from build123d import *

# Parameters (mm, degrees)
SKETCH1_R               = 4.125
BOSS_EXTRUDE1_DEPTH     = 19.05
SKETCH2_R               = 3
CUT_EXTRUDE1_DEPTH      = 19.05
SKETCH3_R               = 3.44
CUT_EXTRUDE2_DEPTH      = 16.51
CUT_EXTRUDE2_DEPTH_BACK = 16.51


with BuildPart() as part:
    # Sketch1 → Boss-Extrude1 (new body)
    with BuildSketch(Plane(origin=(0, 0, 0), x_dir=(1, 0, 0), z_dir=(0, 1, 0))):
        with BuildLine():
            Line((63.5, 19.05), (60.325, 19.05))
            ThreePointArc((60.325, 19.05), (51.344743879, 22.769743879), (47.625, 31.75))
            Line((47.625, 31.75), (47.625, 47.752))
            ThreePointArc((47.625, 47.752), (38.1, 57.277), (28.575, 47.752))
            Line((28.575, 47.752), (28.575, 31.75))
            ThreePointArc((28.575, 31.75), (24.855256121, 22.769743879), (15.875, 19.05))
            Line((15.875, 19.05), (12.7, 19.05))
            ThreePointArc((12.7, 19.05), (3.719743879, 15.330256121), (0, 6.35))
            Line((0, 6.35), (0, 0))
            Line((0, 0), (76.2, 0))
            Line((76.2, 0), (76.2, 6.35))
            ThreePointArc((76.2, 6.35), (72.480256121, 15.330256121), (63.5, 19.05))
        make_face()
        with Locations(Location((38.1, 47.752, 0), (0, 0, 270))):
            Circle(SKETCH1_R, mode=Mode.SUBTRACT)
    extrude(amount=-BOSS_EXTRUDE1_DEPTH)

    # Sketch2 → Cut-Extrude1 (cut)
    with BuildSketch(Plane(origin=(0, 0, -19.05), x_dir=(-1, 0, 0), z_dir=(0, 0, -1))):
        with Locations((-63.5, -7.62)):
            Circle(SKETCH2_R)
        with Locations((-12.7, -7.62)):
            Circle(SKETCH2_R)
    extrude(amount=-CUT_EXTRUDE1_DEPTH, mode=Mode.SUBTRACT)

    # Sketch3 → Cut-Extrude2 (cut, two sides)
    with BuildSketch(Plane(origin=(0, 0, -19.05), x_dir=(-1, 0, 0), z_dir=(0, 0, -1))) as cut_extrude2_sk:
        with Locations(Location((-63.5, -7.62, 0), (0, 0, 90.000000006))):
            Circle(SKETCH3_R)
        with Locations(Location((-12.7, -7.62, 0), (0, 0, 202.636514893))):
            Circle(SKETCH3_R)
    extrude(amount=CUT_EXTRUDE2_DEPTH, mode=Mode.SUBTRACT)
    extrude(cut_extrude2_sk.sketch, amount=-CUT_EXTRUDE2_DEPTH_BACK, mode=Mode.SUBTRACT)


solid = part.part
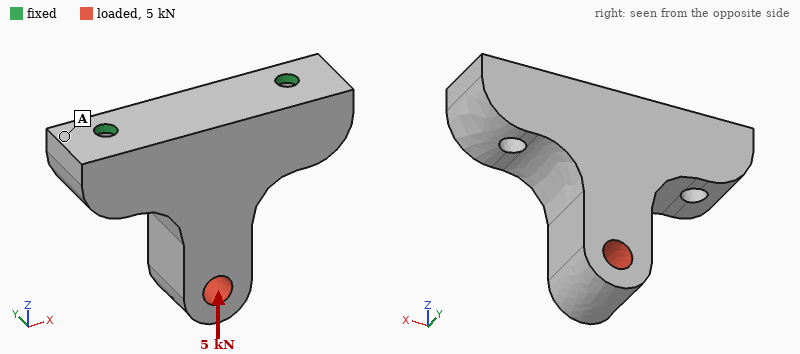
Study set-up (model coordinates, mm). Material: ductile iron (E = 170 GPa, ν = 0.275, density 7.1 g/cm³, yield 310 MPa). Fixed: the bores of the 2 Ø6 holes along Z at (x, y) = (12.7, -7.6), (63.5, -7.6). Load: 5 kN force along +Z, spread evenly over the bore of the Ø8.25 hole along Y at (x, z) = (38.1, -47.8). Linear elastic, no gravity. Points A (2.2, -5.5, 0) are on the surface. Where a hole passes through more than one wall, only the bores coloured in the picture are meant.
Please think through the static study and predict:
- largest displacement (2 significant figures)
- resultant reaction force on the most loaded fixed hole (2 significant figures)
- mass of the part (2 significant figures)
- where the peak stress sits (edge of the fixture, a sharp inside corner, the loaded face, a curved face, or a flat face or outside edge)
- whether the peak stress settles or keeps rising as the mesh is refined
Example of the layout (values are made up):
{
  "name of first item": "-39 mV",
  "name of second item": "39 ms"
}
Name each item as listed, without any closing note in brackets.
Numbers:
{
  "largest displacement": "25 µm",
  "resultant reaction force on the most loaded fixed hole": "2.9 kN",
  "mass of the part": "270 g",
  "where the peak stress sits": "edge of the fixture",
  "whether the peak stress settles or keeps rising as the mesh is refined": "keeps rising"
}
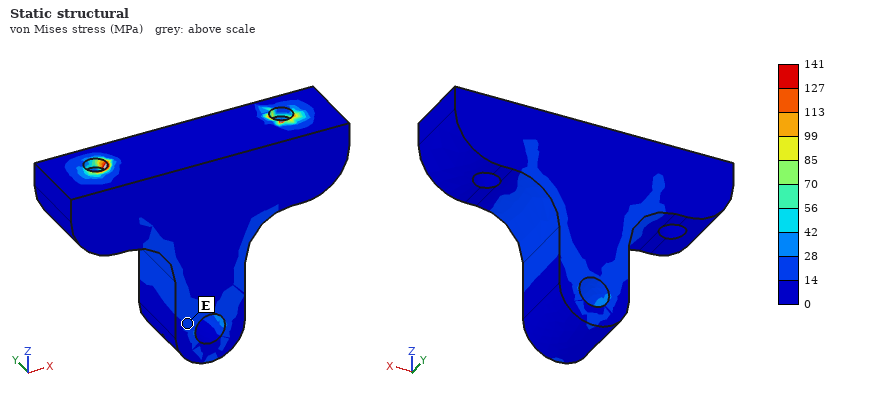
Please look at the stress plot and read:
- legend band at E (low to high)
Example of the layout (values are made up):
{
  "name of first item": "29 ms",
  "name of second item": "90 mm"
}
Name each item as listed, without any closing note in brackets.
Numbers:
{
  "legend band at E": "14 to 28 MPa"
}
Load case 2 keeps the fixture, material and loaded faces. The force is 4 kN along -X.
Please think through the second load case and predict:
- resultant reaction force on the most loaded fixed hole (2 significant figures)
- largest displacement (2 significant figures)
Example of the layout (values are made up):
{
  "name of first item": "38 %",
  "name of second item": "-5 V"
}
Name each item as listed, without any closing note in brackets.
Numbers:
{
  "resultant reaction force on the most loaded fixed hole": "4.2 kN",
  "largest displacement": "39 µm"
}
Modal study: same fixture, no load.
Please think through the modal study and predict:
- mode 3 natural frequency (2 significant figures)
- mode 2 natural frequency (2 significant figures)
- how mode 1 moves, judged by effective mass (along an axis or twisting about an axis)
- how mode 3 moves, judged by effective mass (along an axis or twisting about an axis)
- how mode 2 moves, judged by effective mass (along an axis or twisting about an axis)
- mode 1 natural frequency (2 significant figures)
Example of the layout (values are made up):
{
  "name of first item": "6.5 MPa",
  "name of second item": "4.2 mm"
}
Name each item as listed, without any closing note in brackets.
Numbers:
{
  "mode 3 natural frequency": "12 kHz",
  "mode 2 natural frequency": "8600 Hz",
  "how mode 1 moves, judged by effective mass": "along Y",
  "how mode 3 moves, judged by effective mass": "along Z",
  "how mode 2 moves, judged by effective mass": "along X",
  "mode 1 natural frequency": "2000 Hz"
}
